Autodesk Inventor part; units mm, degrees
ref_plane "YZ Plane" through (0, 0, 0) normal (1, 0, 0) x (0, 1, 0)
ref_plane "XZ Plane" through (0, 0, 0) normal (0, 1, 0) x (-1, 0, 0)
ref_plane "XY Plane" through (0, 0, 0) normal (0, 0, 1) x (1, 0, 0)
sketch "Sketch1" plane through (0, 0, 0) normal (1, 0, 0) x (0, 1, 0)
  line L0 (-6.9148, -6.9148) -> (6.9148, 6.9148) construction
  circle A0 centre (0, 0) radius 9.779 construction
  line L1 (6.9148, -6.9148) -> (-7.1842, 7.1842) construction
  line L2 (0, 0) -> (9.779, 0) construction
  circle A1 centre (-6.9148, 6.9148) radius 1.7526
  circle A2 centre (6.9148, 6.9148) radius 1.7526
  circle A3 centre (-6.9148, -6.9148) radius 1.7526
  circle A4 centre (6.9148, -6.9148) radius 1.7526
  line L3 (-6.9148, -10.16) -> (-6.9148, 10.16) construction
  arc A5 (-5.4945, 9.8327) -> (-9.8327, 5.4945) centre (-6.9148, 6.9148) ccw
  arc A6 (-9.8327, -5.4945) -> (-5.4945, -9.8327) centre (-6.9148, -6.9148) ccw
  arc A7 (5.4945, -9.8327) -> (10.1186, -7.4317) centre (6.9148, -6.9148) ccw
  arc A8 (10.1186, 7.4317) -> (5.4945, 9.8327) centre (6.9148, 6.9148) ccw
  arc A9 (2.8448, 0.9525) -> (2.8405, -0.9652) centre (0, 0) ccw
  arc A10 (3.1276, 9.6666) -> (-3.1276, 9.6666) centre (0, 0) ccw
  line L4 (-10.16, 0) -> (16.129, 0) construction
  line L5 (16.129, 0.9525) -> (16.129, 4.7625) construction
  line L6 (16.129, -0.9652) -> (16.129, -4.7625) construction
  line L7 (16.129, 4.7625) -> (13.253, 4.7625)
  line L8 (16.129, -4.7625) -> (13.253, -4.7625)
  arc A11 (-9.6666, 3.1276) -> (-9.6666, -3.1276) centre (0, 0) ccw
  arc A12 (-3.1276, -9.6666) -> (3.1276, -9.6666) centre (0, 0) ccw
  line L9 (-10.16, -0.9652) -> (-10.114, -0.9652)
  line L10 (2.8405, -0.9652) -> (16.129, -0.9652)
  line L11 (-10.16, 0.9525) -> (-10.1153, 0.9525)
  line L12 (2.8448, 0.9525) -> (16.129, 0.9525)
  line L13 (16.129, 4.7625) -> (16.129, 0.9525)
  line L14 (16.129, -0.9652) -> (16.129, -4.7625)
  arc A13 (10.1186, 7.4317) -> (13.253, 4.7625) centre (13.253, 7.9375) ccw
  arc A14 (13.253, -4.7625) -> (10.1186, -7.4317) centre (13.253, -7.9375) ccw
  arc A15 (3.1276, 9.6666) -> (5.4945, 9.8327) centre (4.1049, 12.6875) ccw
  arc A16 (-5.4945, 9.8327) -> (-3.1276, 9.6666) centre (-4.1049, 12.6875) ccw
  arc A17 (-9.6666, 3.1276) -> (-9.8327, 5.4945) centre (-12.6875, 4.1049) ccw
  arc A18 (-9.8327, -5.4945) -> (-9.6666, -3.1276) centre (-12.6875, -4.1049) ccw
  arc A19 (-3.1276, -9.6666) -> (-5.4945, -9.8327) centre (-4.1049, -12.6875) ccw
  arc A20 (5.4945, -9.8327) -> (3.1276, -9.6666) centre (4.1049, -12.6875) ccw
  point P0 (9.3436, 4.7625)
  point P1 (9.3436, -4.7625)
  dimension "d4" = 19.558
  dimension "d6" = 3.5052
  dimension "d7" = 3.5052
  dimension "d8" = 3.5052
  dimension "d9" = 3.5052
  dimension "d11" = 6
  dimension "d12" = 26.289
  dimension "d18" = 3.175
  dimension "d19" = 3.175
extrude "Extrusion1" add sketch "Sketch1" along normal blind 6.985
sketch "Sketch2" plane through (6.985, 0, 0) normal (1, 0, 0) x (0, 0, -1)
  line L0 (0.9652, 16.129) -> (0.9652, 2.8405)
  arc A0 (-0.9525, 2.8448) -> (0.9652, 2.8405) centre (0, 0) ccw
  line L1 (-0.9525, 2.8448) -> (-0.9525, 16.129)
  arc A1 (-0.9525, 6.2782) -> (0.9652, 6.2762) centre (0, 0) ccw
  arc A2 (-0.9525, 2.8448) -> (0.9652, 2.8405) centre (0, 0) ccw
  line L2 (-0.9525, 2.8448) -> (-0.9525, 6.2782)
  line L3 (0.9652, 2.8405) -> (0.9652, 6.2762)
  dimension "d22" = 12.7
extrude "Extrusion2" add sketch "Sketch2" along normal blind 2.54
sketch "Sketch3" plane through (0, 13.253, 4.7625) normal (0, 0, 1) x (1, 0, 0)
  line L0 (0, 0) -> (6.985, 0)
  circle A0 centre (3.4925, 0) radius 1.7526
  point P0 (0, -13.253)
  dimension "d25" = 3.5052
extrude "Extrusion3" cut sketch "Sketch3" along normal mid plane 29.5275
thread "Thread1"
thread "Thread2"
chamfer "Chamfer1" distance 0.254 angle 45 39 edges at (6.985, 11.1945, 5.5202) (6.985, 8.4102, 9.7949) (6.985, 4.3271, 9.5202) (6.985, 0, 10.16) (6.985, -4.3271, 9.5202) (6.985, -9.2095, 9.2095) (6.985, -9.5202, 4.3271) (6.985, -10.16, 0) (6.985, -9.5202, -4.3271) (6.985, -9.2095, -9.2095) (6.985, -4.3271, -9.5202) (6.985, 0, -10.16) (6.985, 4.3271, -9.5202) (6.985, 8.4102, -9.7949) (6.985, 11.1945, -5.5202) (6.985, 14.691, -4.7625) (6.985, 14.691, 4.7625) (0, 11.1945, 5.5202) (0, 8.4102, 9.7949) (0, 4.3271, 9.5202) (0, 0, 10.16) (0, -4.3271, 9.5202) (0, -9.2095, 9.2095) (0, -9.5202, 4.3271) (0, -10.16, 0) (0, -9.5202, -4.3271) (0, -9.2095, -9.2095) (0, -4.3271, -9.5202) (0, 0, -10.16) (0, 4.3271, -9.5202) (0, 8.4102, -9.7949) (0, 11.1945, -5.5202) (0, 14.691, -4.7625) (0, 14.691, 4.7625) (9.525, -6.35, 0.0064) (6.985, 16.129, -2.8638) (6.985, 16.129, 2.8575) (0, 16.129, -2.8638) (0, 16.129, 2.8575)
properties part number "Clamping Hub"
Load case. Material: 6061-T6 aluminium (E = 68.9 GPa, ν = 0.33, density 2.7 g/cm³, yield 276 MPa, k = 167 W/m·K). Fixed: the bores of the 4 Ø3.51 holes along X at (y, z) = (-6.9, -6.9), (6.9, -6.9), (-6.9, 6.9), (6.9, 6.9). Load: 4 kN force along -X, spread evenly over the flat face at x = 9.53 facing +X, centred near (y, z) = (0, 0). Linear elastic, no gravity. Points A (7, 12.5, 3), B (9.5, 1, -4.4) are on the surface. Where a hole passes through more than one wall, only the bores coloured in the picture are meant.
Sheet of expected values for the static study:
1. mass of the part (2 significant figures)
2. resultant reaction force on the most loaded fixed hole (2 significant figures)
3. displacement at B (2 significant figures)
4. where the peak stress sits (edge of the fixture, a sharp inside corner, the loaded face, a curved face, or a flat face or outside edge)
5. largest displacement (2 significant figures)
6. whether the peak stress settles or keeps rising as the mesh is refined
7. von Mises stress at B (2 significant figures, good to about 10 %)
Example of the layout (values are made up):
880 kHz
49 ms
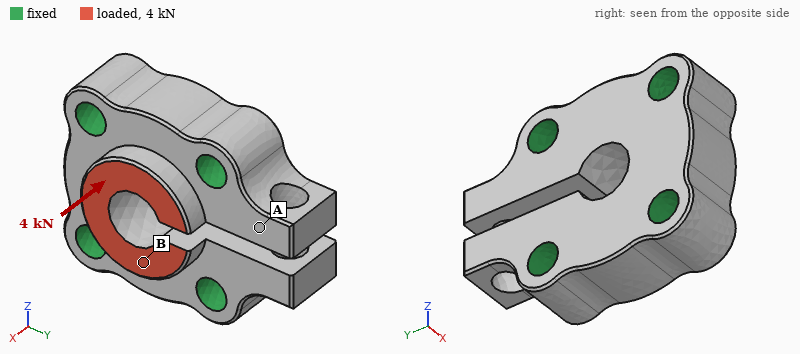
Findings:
7.2 g
1.1 kN
6.7 µm
edge of the fixture
10 µm
keeps rising
41 MPa
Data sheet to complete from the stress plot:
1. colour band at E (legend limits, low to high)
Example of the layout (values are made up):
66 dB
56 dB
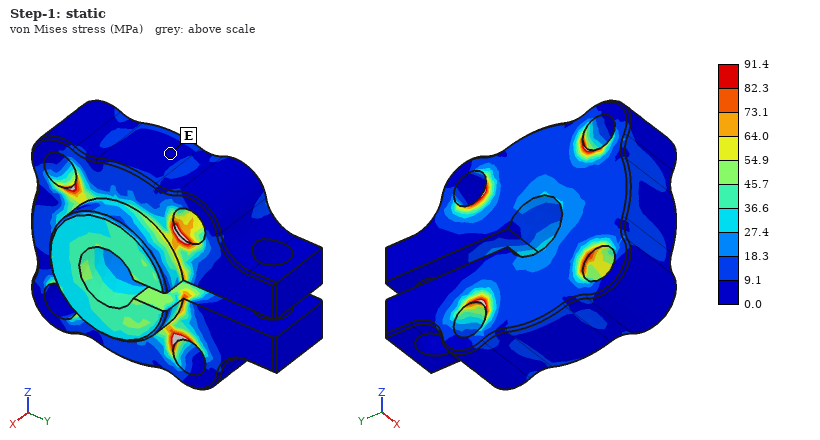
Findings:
0.0 to 9.1 MPa
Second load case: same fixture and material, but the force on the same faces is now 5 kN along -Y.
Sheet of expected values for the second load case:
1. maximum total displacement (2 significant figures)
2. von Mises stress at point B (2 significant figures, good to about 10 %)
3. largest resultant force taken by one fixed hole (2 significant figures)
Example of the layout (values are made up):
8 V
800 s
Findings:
22 µm
120 MPa
1.7 kN
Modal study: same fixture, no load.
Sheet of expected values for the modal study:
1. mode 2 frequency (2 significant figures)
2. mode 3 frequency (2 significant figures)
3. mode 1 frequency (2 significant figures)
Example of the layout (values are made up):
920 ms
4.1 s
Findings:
51 kHz
51 kHz
51 kHz
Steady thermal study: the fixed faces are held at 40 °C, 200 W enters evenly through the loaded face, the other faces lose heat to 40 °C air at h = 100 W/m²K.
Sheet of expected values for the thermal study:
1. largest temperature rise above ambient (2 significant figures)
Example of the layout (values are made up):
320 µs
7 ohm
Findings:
74 K
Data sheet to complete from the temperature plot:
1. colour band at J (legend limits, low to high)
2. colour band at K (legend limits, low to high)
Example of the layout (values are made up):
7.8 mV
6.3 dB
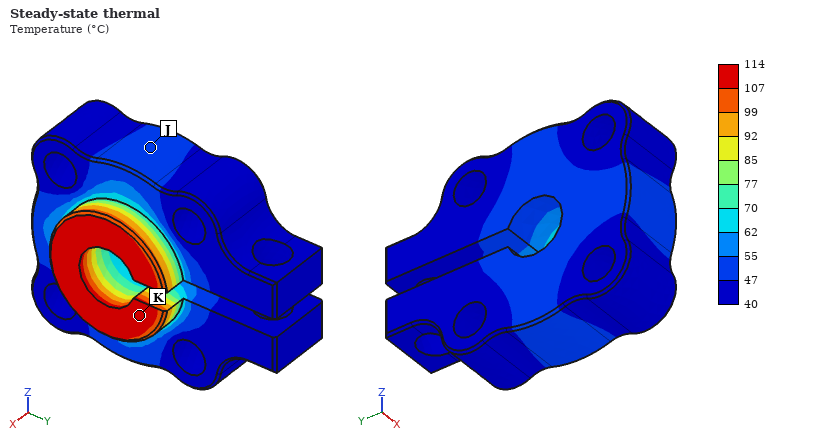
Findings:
47 to 55 °C
107 to 114 °C
